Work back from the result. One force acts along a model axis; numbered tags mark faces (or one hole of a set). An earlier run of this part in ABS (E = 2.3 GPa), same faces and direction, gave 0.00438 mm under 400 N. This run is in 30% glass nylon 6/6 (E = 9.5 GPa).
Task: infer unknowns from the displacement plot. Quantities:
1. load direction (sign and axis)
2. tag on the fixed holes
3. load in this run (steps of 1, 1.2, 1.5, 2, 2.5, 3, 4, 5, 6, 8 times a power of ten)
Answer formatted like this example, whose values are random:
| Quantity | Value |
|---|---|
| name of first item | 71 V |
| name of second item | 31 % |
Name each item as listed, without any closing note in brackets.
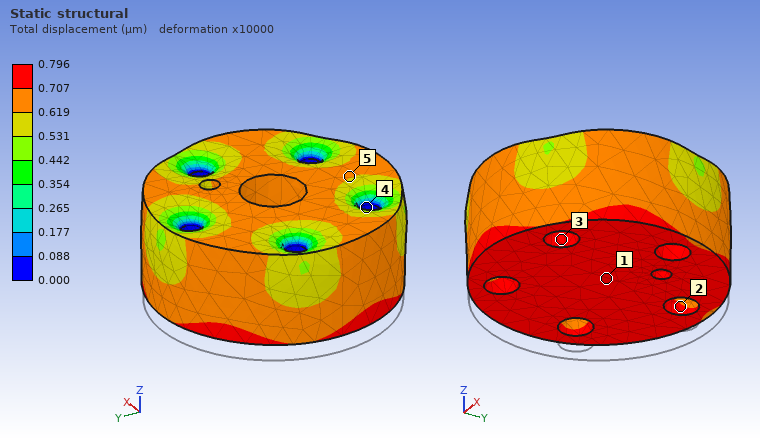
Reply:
| Quantity | Value |
|---|---|
| load direction | +Z |
| tag on the fixed holes | 4 |
| load in this run | 300 N |
